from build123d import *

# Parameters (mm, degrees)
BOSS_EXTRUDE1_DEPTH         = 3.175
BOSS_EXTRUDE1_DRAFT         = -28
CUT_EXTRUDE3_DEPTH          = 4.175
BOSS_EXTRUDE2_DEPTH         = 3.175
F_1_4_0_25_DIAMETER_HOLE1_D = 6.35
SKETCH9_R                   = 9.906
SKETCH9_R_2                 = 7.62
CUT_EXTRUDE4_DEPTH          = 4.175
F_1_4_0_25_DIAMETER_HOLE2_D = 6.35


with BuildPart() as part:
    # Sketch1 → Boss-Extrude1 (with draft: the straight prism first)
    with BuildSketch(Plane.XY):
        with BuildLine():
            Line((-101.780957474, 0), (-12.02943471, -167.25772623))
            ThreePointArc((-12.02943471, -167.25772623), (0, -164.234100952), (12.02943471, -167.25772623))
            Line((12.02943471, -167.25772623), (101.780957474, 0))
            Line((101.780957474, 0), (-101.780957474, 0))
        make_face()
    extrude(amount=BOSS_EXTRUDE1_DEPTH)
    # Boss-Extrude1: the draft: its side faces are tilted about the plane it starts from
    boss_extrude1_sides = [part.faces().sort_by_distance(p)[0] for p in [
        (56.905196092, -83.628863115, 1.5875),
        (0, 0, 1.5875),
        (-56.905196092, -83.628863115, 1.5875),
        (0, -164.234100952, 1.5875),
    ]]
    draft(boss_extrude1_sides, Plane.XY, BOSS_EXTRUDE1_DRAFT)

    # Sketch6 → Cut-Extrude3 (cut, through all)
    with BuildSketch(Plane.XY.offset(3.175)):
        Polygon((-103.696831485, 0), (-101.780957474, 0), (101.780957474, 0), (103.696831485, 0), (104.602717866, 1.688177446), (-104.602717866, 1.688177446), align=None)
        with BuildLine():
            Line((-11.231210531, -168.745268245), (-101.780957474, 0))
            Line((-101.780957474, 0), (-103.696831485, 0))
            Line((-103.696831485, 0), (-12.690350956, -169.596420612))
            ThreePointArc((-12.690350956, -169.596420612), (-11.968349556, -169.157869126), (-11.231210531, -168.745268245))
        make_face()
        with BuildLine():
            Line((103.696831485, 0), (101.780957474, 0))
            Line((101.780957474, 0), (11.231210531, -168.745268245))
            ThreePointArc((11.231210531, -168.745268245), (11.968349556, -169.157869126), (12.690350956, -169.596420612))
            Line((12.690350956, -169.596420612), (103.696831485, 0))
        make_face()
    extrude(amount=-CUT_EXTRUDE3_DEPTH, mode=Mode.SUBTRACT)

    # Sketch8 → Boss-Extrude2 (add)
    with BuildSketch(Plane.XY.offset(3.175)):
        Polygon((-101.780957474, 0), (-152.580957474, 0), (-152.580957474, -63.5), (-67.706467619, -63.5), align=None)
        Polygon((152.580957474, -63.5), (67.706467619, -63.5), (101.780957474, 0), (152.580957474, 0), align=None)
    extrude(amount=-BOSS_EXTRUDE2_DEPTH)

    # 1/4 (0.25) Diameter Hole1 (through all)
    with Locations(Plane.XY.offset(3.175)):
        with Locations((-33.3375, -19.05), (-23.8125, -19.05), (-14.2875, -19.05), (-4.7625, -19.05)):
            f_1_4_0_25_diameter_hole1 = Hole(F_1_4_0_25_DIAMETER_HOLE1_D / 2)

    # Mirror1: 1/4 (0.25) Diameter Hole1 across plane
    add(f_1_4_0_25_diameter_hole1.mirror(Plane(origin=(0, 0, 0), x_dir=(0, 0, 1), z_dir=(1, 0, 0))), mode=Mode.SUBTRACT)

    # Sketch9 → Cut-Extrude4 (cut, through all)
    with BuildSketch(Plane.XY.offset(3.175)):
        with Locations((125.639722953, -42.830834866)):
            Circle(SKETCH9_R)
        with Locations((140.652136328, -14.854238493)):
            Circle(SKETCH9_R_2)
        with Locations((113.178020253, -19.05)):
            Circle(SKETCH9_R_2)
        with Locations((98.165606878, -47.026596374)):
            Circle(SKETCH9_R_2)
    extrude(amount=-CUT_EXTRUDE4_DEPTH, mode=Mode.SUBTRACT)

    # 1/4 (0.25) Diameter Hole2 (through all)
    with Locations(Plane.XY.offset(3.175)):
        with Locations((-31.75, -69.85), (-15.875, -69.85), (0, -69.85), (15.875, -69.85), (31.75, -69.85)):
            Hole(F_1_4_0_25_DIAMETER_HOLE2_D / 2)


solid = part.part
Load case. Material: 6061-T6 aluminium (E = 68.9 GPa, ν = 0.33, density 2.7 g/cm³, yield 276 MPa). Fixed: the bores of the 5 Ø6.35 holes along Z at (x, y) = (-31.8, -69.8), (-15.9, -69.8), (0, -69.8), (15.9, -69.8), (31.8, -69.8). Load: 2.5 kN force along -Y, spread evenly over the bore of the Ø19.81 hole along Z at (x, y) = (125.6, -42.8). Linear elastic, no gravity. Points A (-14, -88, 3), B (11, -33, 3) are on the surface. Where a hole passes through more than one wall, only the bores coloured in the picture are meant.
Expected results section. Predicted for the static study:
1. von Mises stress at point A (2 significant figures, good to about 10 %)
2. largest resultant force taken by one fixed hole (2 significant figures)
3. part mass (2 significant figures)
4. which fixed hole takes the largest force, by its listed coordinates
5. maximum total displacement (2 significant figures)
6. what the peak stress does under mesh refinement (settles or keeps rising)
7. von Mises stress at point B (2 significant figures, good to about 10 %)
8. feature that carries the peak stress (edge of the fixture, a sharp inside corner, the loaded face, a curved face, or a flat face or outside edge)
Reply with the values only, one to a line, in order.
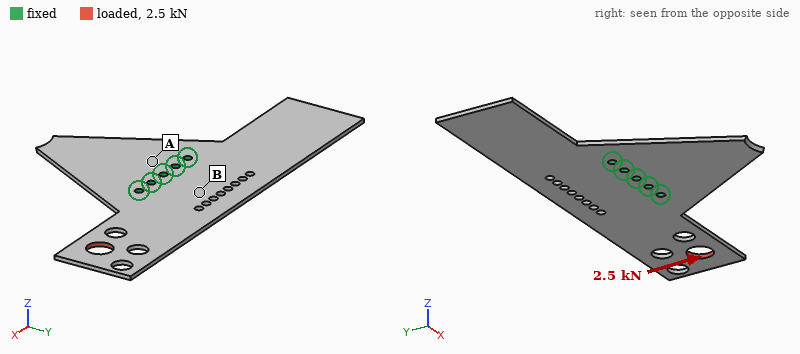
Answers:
14 MPa
5.4 kN
230 g
(31.8, -69.8)
0.40 mm
keeps rising
31 MPa
edge of the fixture
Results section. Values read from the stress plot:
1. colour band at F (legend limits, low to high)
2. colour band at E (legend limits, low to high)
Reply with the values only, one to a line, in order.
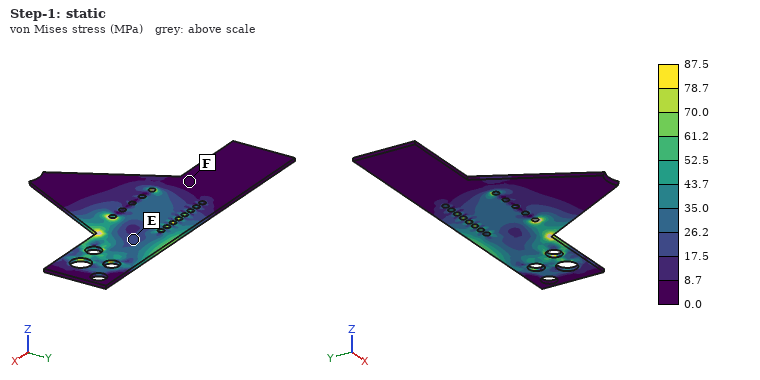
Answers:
0.0 to 8.7 MPa
17.5 to 26.2 MPa
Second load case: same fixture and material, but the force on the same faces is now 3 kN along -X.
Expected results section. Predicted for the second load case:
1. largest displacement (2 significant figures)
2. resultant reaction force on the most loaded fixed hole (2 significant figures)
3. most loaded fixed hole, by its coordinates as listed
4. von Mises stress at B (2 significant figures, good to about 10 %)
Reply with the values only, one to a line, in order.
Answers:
54 µm
1.7 kN
(31.8, -69.8)
12 MPa
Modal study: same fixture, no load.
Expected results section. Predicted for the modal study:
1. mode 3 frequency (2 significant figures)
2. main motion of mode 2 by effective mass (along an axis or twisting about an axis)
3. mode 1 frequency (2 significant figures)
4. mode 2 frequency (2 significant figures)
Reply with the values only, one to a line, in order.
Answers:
430 Hz
along Z
160 Hz
180 Hz
